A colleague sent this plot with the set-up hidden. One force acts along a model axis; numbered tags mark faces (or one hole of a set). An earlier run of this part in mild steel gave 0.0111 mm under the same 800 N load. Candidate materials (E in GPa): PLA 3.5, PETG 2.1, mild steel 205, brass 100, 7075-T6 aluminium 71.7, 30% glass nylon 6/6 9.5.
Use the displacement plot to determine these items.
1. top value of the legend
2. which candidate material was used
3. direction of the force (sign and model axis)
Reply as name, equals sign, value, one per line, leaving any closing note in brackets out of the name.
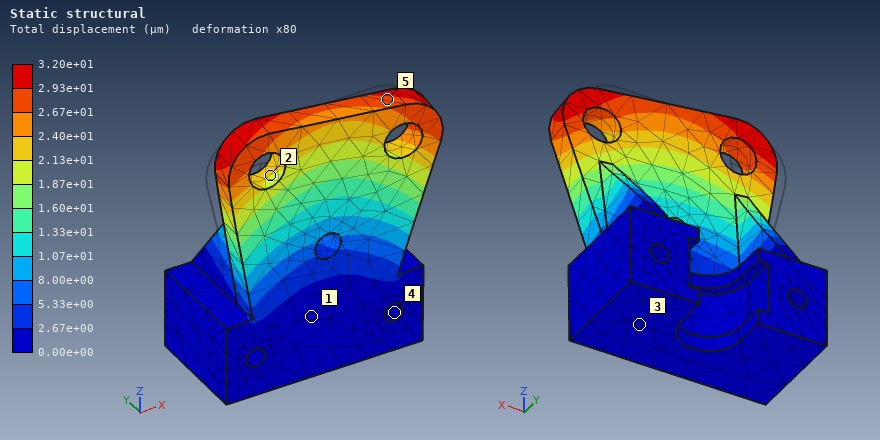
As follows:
top value of the legend = 3.20e+01 µm
which candidate material was used = 7075-T6 aluminium
direction of the force = +X
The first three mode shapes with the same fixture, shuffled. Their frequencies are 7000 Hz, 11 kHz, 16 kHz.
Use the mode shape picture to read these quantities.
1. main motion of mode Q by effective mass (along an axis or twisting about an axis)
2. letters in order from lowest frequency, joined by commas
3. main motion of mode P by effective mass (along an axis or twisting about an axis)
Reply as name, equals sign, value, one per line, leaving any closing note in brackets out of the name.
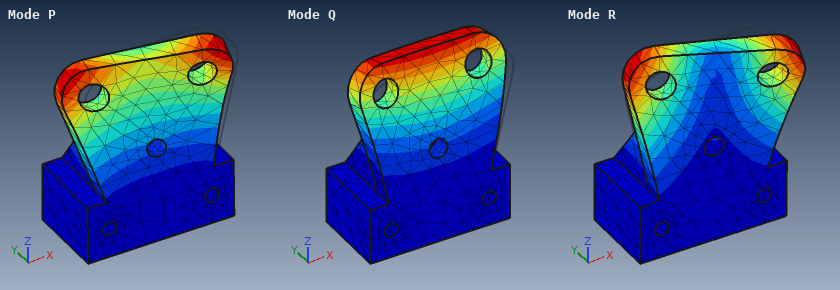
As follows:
main motion of mode Q by effective mass = along Y
letters in order from lowest frequency, joined by commas = Q, R, P
main motion of mode P by effective mass = along X
